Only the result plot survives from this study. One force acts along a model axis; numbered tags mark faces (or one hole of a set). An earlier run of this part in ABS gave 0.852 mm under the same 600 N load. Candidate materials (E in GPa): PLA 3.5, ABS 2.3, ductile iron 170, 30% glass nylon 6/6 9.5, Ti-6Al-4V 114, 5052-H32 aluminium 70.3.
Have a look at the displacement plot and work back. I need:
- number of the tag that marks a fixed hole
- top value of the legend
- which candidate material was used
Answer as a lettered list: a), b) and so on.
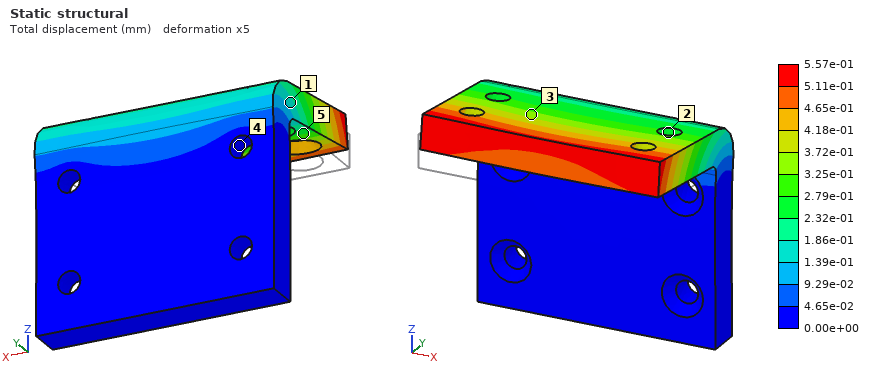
a) 4
b) 5.57e-01 mm
c) PLA
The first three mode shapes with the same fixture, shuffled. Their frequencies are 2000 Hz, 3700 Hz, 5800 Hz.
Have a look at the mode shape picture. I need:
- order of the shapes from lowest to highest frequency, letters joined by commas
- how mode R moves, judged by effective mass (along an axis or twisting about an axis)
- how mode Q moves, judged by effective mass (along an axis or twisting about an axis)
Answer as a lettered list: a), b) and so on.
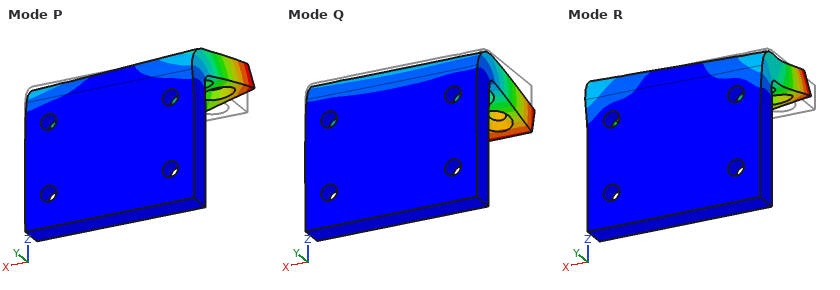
a) Q, P, R
b) along X
c) along Z
